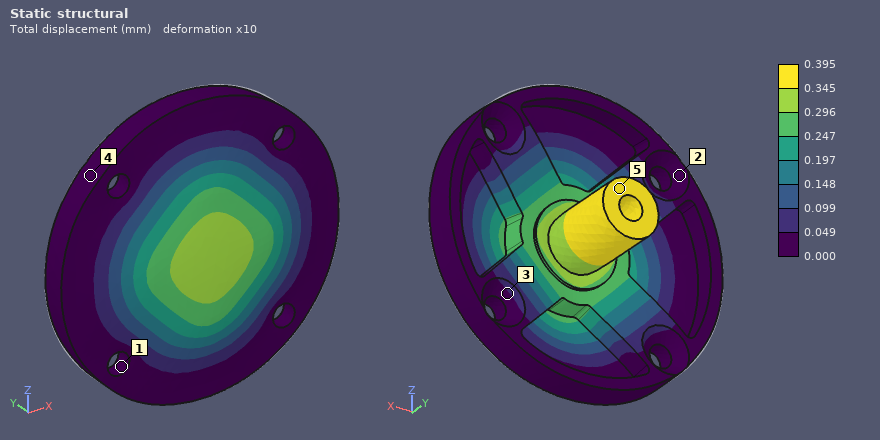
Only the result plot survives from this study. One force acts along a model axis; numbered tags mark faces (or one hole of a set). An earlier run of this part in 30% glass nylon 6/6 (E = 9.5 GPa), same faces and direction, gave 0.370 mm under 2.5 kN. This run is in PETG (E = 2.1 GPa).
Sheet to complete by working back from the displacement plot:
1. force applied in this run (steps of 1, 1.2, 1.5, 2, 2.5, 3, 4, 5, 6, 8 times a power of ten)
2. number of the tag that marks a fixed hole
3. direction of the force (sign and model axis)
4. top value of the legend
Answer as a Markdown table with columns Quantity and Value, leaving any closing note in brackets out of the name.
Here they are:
| Quantity | Value |
|---|---|
| force applied in this run | 600 N |
| number of the tag that marks a fixed hole | 1 |
| direction of the force | -Y |
| top value of the legend | 0.395 mm |
